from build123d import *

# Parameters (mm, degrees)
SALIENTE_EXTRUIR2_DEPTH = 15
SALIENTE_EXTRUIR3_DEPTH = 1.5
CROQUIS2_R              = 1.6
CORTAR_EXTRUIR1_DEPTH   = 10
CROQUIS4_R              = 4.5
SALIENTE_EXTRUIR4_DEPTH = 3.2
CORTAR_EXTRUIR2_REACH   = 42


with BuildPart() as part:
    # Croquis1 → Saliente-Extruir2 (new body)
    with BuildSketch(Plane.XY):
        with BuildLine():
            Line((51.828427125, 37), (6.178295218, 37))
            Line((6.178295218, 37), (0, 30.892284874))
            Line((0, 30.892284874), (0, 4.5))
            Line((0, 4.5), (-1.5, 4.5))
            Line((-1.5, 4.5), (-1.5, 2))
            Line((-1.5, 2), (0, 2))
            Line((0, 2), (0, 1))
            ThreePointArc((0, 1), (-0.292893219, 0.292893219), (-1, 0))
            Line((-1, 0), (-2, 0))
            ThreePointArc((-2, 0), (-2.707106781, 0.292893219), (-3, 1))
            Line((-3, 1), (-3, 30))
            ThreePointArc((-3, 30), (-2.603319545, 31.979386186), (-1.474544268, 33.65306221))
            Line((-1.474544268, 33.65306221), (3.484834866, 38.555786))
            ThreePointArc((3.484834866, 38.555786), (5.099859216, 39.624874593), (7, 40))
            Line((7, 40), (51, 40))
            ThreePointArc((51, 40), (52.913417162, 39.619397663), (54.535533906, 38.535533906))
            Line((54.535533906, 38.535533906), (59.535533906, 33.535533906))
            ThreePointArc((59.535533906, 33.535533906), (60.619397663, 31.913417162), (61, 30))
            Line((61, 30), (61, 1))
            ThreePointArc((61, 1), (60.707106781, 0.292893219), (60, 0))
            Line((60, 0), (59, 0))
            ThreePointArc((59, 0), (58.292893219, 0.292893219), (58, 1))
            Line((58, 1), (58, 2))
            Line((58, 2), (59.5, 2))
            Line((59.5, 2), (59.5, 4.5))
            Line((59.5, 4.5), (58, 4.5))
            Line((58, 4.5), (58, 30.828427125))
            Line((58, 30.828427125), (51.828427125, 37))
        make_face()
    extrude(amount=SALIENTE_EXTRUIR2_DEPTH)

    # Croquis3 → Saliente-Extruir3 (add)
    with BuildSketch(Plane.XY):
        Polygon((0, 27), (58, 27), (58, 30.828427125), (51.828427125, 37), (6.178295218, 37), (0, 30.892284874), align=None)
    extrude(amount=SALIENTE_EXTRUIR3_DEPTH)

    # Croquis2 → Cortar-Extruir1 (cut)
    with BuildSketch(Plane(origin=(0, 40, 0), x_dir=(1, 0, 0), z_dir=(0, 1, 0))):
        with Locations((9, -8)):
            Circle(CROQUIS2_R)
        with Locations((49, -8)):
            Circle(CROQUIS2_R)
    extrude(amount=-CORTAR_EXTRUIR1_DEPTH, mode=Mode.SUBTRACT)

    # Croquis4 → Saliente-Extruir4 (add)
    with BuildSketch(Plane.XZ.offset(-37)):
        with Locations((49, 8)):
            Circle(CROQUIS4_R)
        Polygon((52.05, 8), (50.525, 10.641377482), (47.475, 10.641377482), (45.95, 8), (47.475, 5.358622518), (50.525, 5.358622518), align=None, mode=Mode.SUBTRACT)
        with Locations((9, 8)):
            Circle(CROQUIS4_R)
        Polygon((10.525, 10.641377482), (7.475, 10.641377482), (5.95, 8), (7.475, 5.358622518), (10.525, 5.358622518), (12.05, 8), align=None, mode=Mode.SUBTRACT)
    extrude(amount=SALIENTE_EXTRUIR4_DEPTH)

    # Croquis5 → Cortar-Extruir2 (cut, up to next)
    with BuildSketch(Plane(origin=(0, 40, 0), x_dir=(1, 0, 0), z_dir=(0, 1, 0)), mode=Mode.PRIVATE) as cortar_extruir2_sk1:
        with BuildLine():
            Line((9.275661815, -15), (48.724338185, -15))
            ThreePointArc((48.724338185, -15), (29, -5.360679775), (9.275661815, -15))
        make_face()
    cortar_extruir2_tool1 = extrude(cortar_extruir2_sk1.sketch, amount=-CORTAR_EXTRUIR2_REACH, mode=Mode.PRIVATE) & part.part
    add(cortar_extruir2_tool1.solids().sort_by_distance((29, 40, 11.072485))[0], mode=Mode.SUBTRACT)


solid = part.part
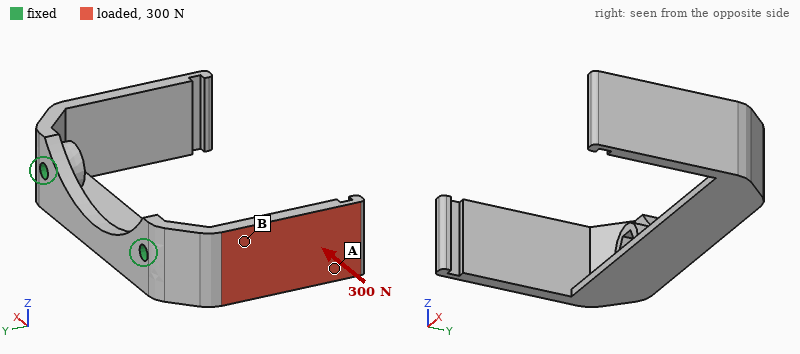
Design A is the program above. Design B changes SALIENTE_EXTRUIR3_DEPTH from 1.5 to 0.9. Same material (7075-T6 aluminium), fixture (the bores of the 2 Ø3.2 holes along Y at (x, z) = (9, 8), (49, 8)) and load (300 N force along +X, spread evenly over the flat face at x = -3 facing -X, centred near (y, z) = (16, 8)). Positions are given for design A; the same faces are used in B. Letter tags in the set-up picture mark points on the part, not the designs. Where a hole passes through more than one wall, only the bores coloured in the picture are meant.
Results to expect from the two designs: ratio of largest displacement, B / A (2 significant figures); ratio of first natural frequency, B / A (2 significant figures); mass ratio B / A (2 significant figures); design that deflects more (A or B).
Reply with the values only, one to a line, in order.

1.1
0.94
0.94
B
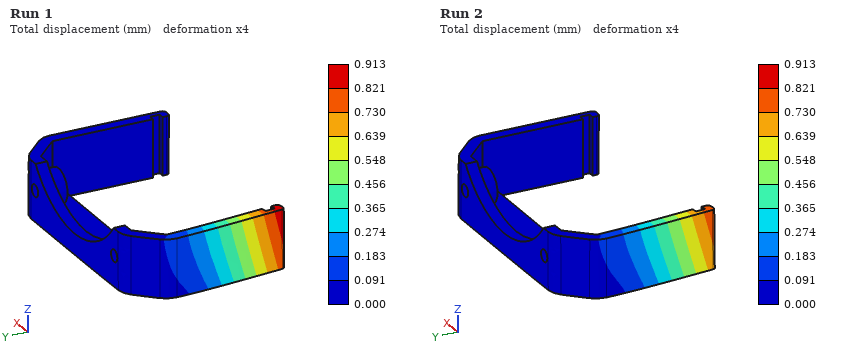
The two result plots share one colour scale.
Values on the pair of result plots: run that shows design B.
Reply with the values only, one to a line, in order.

Run 1
